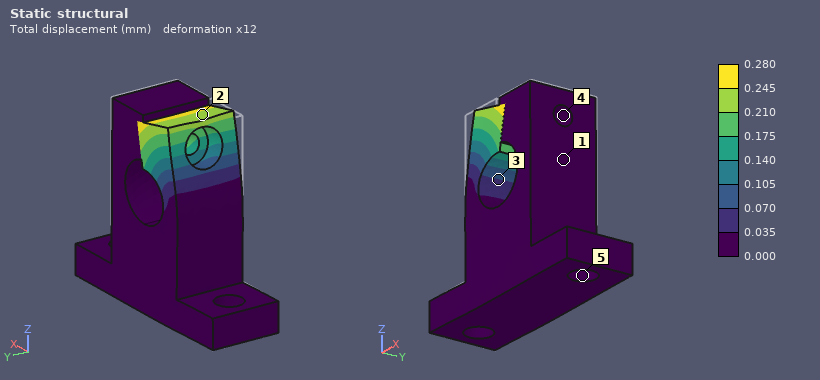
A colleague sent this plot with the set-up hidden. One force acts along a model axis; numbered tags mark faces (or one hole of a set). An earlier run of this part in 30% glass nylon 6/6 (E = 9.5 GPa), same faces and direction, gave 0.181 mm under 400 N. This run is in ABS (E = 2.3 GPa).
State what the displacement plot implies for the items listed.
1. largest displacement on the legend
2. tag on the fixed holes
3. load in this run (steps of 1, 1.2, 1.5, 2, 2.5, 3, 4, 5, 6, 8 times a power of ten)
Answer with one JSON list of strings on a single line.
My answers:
["0.280 mm", "5", "150 N"]
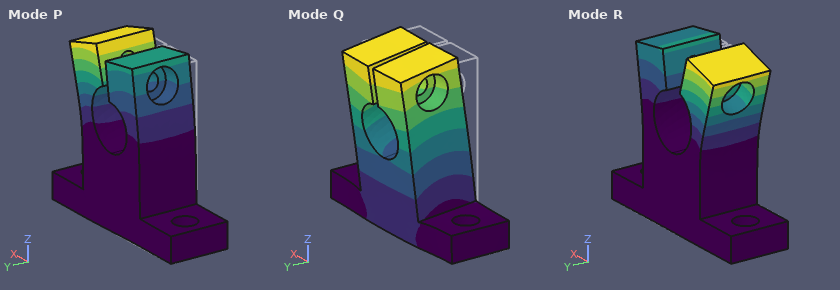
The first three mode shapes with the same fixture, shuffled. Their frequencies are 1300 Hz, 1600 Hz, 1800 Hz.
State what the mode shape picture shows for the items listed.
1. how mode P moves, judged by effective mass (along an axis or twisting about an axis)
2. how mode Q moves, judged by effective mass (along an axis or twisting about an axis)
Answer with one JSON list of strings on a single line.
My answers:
["along X", "along Y"]
